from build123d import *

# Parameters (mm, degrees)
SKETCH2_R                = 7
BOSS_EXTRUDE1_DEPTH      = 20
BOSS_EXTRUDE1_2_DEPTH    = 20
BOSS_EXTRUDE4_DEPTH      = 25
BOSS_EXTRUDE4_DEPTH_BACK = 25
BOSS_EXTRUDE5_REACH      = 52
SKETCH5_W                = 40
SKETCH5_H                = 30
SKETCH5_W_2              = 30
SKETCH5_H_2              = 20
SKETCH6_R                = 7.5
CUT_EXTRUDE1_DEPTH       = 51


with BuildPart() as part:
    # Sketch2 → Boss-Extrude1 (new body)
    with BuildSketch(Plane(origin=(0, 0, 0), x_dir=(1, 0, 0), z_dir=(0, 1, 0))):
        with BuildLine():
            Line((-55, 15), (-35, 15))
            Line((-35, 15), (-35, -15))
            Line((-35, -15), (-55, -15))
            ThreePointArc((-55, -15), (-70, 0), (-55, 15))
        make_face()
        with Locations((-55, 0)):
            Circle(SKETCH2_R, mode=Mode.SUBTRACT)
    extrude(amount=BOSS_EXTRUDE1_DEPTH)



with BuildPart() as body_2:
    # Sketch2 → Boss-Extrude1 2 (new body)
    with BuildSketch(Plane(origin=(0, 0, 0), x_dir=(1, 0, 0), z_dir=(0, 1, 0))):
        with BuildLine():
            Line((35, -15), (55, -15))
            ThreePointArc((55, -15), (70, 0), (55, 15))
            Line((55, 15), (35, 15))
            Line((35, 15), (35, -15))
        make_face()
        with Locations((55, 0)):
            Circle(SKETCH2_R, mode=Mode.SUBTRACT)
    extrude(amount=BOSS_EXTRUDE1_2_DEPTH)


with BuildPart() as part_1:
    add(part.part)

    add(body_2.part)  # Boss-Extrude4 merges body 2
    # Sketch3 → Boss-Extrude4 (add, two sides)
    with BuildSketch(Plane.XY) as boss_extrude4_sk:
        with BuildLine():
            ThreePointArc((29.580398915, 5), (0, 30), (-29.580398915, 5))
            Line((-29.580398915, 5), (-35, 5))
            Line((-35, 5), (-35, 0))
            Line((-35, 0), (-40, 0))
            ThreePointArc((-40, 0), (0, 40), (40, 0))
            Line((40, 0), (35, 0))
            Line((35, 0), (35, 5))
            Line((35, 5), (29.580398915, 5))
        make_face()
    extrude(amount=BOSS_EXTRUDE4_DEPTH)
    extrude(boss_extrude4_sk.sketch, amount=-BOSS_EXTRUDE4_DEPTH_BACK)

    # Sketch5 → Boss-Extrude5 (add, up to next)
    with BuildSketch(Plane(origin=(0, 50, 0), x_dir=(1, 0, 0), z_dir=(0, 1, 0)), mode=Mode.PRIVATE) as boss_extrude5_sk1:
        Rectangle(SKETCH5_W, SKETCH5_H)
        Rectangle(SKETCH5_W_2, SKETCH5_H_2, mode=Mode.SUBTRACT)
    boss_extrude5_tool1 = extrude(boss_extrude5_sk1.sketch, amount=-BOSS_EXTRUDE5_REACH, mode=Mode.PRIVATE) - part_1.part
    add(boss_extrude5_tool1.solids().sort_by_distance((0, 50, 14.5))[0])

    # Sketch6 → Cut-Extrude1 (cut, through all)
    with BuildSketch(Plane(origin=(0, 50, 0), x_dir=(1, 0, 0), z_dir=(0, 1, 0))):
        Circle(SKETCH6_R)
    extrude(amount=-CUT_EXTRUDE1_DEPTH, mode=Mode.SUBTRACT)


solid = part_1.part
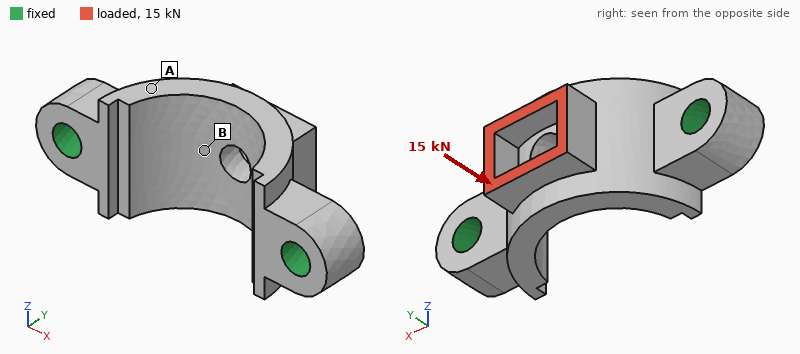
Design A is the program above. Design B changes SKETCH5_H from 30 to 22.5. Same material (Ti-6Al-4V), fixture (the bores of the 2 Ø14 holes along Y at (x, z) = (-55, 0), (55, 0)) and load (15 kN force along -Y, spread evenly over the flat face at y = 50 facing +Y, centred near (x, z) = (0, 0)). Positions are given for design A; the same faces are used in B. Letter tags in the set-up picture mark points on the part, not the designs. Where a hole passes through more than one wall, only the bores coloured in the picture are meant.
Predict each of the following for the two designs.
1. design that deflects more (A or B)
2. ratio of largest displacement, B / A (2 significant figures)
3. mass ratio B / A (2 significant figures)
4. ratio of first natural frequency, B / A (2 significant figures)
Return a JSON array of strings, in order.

["B", "1.2", "0.96", "1.1"]
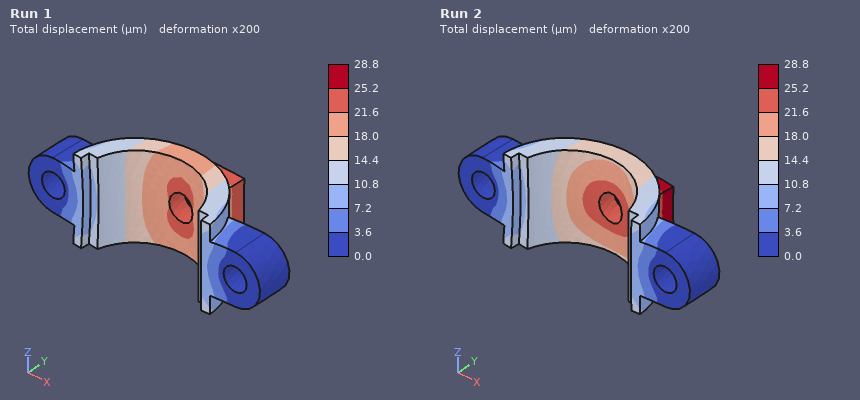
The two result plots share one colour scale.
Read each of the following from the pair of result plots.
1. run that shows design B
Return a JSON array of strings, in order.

["Run 2"]
